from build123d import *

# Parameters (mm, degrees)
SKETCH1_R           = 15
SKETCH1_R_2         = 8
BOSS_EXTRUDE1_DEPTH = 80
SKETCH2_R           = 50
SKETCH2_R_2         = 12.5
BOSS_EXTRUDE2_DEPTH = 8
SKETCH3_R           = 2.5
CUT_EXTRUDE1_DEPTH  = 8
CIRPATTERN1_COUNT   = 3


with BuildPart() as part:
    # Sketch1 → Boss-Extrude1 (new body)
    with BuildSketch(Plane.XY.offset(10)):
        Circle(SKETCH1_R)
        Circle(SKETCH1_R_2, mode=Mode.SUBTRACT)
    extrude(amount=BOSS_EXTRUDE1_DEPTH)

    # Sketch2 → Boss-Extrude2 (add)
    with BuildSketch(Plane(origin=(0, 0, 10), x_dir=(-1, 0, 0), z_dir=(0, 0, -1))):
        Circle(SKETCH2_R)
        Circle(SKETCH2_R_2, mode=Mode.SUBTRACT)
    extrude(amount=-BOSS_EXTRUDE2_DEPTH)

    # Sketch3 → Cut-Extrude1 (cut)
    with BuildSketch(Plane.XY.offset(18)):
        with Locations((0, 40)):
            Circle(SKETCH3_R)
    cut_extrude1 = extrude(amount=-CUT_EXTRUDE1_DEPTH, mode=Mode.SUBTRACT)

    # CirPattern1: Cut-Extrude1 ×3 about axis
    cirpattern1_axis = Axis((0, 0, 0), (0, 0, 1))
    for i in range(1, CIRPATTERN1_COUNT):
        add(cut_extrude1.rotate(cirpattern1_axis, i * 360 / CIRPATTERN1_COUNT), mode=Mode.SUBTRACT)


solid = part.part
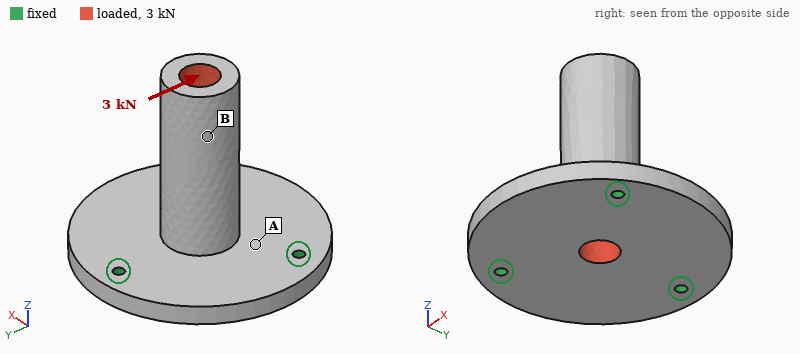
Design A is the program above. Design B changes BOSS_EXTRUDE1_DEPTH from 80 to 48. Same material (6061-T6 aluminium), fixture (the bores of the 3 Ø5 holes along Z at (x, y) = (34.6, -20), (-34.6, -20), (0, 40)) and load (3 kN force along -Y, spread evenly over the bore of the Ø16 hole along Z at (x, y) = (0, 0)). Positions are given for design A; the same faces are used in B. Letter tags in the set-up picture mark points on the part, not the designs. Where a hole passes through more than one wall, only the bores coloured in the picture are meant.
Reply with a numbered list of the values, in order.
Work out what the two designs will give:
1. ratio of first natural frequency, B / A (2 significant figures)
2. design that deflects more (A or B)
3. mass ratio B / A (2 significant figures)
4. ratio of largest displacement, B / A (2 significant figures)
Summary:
1. 2.0
2. A
3. 0.83
4. 0.31
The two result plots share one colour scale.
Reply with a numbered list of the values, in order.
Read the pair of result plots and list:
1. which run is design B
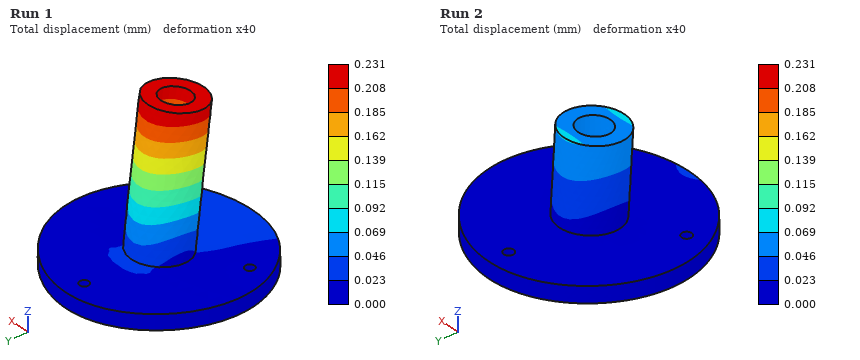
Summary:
1. Run 2
